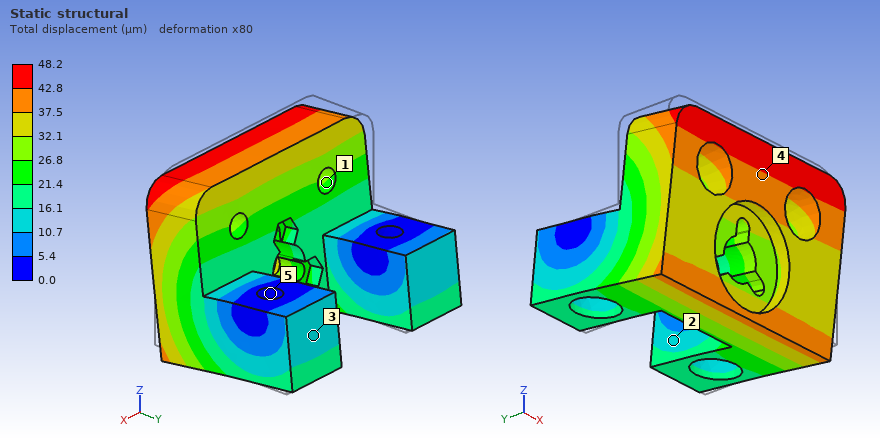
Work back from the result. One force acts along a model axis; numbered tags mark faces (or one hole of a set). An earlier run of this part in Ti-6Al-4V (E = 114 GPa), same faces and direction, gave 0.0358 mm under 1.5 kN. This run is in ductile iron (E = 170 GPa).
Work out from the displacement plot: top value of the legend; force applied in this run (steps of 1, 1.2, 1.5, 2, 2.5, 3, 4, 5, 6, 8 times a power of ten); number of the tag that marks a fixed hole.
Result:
48.2 µm
3 kN
5
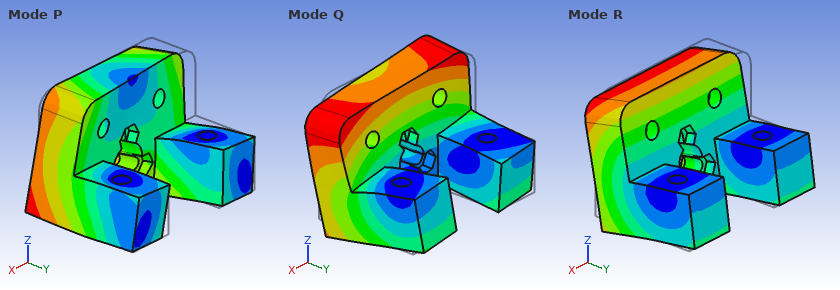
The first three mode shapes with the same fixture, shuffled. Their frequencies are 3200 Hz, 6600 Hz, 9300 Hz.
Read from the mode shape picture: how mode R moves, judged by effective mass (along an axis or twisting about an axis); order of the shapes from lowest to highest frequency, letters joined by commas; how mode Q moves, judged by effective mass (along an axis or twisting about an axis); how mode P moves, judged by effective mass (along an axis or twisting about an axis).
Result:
along Z
R, Q, P
along X
along X
